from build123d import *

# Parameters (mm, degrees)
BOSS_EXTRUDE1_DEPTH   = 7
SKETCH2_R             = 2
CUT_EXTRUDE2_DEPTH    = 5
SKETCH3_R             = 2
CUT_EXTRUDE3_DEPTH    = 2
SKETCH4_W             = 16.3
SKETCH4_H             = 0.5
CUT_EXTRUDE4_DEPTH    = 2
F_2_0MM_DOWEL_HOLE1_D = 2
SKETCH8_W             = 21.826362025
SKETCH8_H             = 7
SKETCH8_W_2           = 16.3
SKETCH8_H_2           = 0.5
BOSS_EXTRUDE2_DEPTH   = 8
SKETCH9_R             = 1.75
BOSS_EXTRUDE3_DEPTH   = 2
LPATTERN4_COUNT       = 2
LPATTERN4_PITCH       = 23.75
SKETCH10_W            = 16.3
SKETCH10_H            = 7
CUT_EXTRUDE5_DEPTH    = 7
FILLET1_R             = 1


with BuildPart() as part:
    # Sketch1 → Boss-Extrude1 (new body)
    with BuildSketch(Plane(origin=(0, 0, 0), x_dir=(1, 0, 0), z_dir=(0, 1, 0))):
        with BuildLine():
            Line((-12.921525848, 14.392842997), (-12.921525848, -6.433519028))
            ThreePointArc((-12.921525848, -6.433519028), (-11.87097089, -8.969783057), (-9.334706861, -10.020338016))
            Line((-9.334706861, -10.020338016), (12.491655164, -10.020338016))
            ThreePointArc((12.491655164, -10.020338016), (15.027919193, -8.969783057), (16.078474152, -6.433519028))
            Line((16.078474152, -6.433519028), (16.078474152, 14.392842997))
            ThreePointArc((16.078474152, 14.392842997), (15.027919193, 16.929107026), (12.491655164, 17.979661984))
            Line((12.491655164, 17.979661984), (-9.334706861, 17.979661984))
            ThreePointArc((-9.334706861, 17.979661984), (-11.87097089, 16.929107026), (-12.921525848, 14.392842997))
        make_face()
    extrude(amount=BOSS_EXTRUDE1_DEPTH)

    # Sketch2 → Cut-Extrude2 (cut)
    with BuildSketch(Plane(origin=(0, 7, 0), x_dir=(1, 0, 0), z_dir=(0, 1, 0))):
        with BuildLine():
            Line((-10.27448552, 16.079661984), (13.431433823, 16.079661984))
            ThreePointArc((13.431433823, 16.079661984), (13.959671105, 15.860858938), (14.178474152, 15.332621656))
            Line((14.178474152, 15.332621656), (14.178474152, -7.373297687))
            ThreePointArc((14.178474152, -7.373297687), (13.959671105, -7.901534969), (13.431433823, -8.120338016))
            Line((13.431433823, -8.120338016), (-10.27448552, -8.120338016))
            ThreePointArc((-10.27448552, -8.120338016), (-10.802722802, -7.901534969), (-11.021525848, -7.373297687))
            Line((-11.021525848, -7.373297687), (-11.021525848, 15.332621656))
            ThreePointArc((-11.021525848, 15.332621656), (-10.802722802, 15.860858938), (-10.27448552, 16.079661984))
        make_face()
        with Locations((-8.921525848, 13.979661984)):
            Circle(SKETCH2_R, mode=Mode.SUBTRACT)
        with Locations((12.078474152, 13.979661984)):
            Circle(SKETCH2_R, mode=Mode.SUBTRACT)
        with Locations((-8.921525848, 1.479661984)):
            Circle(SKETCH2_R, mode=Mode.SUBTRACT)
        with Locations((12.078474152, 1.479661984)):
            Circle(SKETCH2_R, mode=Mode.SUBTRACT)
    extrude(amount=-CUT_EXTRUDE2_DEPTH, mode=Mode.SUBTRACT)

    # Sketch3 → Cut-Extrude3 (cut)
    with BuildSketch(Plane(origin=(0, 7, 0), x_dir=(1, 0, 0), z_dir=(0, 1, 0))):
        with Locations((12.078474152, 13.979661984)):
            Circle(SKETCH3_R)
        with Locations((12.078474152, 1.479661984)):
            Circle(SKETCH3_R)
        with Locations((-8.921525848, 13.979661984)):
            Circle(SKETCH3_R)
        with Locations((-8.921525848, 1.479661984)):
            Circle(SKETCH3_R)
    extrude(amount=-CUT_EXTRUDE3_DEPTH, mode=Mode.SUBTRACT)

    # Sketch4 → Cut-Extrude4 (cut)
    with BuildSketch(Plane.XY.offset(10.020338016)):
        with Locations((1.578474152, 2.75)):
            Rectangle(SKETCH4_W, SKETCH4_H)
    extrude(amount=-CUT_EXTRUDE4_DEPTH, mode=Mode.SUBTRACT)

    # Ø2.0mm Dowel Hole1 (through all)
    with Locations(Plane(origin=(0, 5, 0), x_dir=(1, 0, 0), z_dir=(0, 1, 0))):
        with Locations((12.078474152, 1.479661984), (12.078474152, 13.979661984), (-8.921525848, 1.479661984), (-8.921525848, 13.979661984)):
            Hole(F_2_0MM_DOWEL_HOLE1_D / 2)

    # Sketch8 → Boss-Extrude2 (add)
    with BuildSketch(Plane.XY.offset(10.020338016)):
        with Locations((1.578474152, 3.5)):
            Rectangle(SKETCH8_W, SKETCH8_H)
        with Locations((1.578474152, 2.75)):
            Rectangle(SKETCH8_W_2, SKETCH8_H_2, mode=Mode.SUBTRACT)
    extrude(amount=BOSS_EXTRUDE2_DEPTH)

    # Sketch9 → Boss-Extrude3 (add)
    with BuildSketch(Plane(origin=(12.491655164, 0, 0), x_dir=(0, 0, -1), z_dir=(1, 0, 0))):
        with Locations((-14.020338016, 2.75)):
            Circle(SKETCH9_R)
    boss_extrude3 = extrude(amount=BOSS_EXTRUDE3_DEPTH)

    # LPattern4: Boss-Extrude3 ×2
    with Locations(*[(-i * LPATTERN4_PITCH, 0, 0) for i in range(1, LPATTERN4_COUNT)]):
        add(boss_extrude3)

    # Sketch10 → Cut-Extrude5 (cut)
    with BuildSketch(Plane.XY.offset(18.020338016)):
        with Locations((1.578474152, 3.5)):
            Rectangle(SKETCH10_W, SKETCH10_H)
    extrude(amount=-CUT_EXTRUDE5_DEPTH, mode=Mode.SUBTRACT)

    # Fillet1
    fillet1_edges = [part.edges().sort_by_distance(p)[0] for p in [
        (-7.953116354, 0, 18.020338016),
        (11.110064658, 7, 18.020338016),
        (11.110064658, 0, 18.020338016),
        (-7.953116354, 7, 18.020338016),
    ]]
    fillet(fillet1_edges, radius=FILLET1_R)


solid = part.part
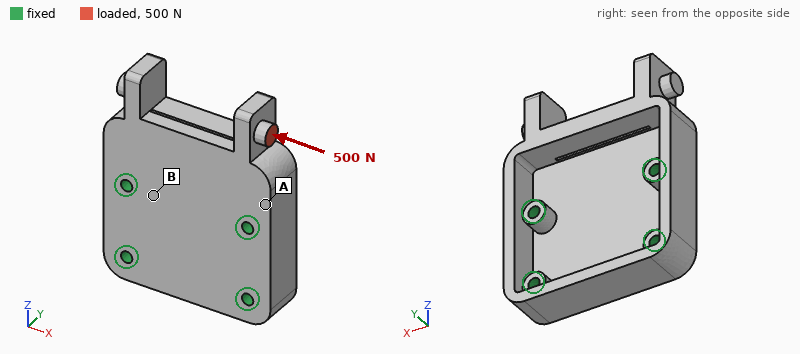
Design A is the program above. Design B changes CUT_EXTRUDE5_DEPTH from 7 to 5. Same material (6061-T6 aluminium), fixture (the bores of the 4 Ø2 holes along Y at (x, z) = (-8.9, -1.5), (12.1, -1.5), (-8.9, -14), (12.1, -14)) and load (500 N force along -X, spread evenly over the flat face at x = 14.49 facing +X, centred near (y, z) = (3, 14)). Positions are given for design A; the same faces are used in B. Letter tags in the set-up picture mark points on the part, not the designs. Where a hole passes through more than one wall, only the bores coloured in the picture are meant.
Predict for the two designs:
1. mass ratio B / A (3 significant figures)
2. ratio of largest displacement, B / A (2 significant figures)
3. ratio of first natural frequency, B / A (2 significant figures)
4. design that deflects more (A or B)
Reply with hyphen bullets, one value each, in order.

- 1.07
- 0.42
- 0.91
- A
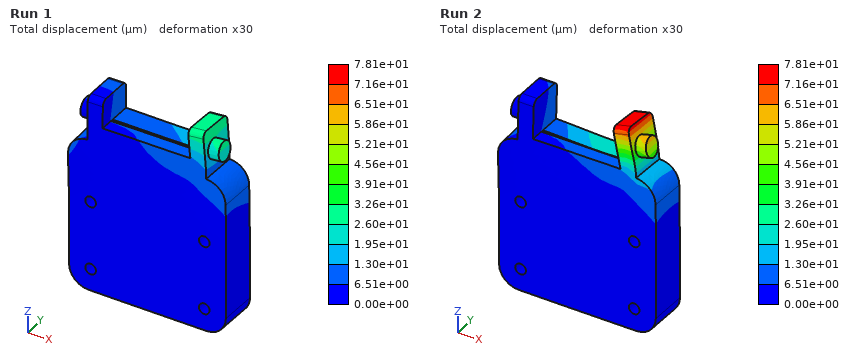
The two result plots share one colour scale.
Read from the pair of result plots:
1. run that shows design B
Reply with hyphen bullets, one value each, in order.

- Run 1
